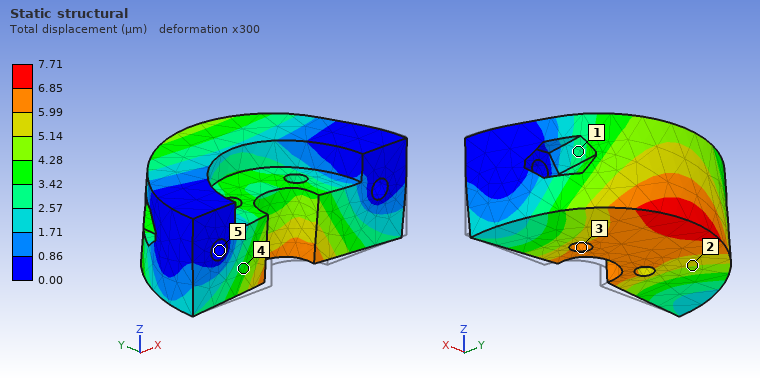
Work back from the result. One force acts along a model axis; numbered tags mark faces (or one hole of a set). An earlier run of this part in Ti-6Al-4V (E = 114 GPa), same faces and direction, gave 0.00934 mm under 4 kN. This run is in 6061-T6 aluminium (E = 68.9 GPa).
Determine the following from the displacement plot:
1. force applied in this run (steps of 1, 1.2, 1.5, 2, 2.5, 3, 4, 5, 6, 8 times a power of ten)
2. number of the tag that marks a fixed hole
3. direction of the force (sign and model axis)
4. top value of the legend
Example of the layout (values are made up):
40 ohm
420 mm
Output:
2 kN
5
+Y
7.71 µm
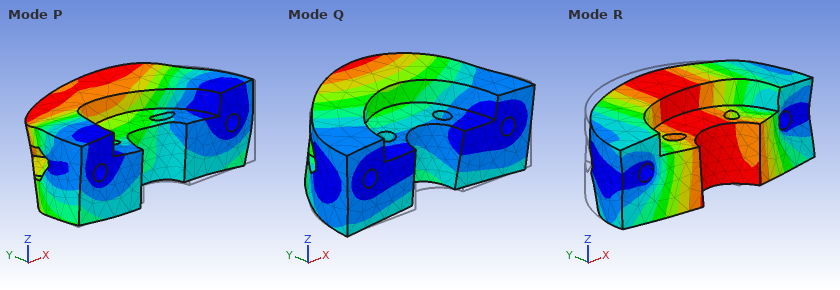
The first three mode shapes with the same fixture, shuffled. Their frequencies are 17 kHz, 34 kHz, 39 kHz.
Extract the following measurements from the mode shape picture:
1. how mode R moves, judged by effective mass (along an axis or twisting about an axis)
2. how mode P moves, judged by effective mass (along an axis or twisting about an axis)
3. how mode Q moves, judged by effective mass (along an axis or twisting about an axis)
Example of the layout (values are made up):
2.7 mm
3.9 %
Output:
along Y
along X
along Z
